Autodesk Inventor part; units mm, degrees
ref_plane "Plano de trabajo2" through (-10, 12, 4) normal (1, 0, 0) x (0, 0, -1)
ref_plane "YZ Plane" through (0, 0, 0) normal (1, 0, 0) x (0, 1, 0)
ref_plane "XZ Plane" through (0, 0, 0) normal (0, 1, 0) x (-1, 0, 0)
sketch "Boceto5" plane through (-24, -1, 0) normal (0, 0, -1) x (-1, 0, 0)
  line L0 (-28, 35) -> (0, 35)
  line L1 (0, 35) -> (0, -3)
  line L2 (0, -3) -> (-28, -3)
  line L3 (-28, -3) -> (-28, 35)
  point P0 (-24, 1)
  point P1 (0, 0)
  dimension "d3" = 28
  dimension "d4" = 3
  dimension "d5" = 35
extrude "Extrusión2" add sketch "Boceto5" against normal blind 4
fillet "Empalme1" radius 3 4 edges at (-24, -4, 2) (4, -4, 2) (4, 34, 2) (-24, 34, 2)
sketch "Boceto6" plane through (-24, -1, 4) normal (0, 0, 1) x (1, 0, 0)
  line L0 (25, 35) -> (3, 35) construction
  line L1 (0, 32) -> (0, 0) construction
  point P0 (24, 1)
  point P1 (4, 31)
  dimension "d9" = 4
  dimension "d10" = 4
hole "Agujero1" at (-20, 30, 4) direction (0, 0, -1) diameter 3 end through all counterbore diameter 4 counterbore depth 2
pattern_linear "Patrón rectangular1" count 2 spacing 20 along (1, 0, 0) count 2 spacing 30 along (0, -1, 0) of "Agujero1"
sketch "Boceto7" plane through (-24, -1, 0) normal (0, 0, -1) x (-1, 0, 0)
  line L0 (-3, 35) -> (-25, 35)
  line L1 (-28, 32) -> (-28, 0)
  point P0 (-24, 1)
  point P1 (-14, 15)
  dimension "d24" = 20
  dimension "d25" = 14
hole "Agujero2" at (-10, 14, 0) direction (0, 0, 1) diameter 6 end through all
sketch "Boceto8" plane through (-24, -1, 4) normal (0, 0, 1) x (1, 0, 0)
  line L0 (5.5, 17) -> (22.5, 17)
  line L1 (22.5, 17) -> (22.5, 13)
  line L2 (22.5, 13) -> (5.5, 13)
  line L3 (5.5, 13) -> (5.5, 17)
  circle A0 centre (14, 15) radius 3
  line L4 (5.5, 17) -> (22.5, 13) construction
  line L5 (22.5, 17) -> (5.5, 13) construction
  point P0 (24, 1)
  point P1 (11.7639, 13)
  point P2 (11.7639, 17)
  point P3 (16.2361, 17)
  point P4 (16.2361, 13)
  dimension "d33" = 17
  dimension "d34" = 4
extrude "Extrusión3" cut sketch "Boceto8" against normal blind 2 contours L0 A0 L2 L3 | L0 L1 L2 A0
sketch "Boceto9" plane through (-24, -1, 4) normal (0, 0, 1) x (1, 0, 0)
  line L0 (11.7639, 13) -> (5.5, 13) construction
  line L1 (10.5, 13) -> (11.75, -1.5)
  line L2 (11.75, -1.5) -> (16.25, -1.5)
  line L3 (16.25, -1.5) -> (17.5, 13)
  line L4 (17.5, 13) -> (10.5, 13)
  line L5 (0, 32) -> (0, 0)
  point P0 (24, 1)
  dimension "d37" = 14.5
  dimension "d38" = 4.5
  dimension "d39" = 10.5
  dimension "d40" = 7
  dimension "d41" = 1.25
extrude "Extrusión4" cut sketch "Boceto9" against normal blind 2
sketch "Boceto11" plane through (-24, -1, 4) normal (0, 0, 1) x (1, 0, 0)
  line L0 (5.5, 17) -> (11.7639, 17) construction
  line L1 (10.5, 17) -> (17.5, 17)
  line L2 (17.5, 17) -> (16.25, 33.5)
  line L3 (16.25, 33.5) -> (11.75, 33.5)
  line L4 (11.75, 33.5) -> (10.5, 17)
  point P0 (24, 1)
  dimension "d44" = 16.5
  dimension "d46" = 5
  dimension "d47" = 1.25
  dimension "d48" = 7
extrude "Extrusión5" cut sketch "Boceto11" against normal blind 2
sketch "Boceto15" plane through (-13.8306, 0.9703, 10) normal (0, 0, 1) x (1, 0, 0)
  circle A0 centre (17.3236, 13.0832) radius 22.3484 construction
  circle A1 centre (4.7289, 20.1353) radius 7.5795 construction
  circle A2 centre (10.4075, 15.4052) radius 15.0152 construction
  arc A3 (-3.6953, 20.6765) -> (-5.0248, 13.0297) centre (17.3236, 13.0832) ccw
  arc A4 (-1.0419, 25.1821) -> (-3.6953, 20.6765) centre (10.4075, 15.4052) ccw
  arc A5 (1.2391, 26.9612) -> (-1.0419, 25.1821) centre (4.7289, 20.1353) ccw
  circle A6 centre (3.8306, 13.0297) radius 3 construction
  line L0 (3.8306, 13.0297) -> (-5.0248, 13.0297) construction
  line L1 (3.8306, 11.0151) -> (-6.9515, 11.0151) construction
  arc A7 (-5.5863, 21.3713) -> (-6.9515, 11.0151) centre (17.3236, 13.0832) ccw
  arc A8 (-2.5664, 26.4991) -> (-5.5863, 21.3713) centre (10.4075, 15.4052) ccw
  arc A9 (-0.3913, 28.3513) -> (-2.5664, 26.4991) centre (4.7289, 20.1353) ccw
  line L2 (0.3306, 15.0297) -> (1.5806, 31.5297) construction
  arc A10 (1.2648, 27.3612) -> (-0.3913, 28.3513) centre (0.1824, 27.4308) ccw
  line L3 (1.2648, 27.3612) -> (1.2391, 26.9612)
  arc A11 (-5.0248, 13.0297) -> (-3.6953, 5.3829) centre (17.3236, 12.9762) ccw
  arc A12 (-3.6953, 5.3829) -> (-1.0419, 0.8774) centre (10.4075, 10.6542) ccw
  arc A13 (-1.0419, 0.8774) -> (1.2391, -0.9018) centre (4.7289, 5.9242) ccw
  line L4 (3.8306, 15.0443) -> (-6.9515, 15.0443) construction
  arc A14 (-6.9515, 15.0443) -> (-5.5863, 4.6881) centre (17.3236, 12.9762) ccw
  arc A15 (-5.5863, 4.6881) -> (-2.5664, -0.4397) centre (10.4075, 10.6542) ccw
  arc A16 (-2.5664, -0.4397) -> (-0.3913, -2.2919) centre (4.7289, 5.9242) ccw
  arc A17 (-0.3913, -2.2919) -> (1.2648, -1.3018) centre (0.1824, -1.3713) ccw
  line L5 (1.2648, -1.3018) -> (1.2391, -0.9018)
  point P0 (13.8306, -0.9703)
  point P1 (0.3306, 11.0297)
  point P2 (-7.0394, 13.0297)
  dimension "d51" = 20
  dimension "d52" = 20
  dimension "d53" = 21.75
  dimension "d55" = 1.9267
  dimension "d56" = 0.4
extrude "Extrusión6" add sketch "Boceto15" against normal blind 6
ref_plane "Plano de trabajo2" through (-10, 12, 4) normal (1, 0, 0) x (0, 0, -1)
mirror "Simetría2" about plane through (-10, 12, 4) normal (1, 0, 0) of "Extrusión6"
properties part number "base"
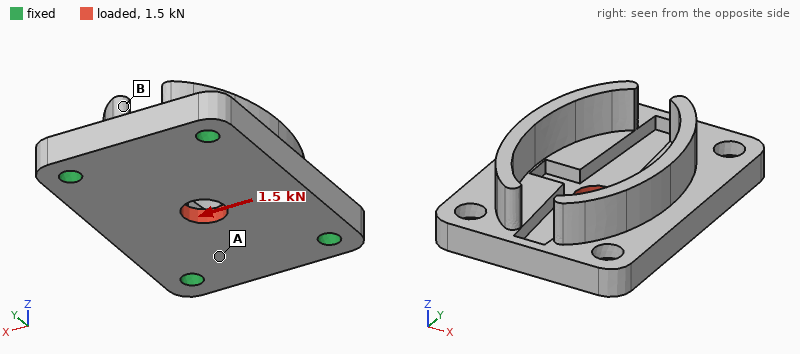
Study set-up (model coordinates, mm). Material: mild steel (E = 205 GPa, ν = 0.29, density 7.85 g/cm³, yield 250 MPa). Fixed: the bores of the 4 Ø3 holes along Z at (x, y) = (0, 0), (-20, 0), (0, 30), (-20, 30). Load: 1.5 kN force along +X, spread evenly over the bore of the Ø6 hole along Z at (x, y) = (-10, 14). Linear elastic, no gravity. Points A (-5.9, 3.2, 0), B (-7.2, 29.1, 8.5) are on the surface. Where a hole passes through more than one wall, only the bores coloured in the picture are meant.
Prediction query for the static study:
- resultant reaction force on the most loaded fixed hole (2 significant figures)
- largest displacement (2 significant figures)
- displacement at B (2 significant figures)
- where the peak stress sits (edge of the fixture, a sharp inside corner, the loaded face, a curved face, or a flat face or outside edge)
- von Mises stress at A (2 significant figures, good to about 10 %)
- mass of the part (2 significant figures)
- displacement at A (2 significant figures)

440 N
2.9 µm
0.57 µm
edge of the fixture
20 MPa
34 g
0.67 µm
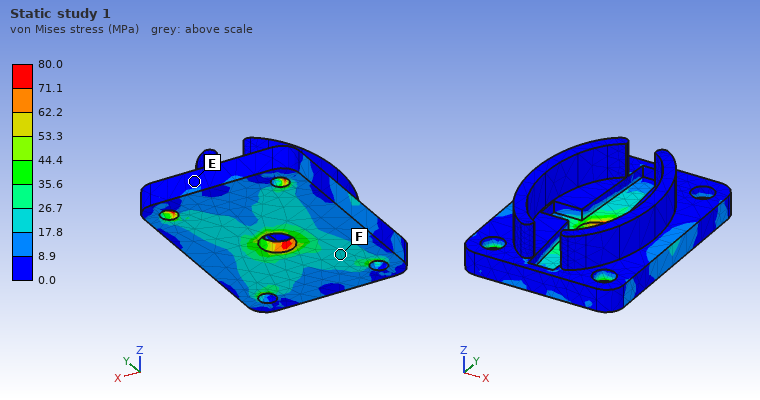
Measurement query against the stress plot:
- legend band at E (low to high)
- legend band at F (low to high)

0.0 to 8.9 MPa
17.8 to 26.7 MPa
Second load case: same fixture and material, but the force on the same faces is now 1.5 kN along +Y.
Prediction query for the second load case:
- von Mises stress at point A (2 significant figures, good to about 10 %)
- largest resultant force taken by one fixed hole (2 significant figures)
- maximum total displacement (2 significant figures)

17 MPa
410 N
1.9 µm
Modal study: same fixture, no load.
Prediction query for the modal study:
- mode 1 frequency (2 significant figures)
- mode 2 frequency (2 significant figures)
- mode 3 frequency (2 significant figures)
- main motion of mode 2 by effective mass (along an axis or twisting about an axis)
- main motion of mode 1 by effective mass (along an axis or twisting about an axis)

18 kHz
20 kHz
21 kHz
along Z
along Z
